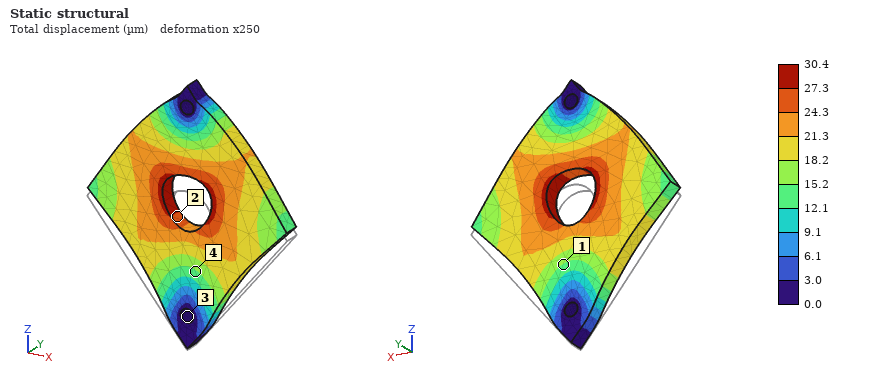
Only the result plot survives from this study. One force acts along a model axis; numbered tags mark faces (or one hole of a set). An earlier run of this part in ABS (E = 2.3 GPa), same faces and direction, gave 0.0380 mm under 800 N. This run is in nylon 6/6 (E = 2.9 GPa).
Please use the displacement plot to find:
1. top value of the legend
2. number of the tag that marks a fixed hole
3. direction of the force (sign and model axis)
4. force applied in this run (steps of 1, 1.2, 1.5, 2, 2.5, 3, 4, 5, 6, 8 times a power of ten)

30.4 µm
3
+Z
800 N
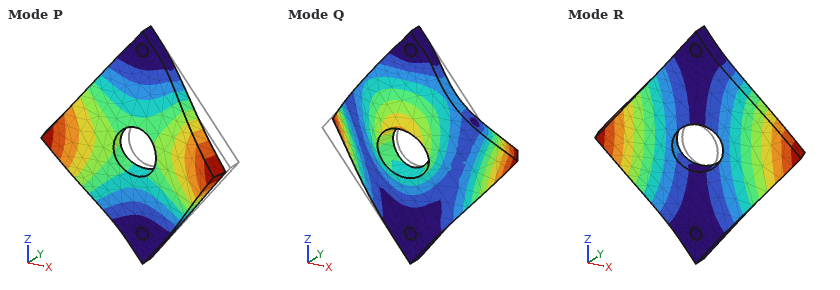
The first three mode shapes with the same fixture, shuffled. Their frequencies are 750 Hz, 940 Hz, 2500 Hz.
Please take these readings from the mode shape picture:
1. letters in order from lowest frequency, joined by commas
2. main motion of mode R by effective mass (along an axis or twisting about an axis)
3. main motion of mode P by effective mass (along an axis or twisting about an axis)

R, P, Q
twisting about Z
along Y
